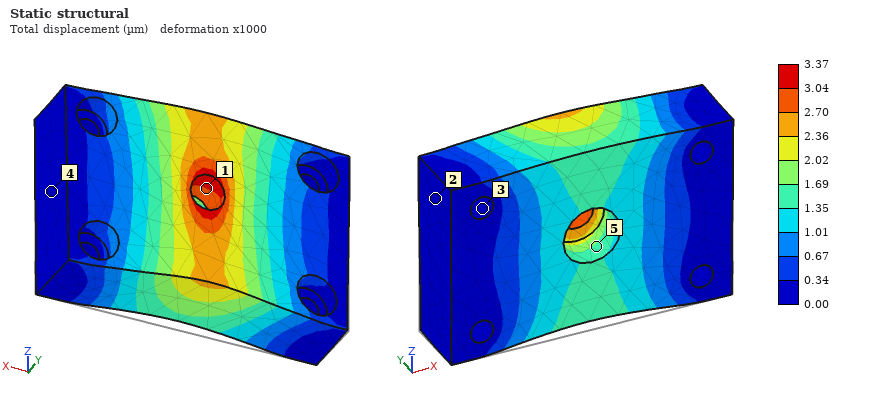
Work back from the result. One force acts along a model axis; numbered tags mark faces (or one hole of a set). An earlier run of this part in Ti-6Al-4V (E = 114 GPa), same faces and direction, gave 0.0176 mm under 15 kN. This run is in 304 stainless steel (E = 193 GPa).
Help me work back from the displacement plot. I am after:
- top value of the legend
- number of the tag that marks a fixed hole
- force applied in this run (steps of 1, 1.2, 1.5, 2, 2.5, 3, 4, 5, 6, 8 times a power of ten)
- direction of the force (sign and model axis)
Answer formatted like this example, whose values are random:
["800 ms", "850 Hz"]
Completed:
["3.37 µm", "3", "5 kN", "+Z"]
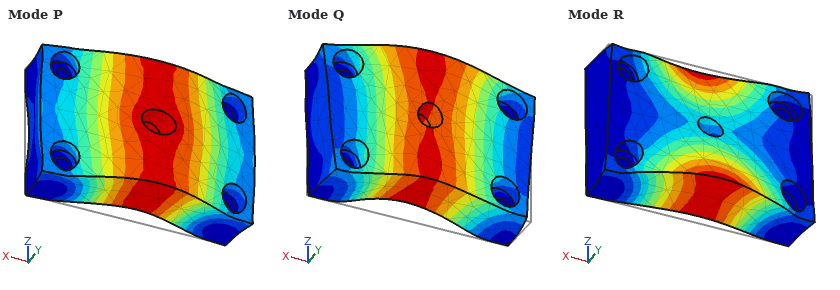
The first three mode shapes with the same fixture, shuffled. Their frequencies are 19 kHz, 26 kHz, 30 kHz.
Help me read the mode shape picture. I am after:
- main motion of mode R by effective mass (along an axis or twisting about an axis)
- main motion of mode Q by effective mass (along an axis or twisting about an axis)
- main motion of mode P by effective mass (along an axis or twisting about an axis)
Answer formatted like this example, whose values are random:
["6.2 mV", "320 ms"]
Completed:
["twisting about X", "along Z", "along Y"]
